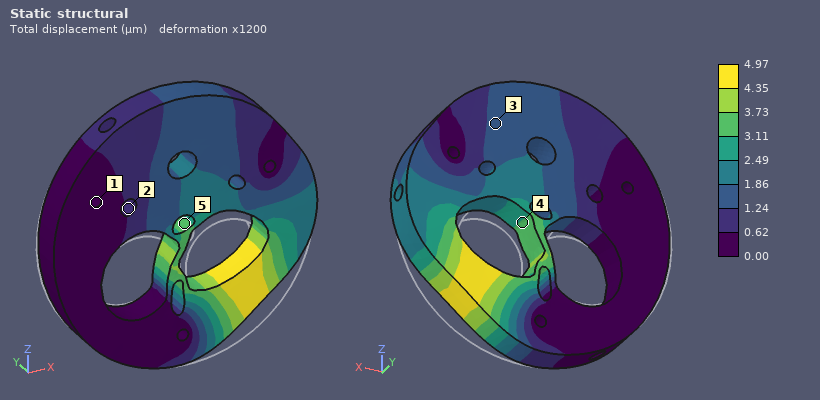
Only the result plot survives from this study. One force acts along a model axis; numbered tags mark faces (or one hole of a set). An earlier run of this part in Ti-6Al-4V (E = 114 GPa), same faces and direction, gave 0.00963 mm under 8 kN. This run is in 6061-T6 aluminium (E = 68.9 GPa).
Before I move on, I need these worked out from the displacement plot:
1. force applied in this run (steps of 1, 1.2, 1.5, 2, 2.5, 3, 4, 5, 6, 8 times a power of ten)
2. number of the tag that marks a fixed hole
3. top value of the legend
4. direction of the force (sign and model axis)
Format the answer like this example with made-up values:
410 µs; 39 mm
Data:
2.5 kN; 1; 4.97 µm; +Z
